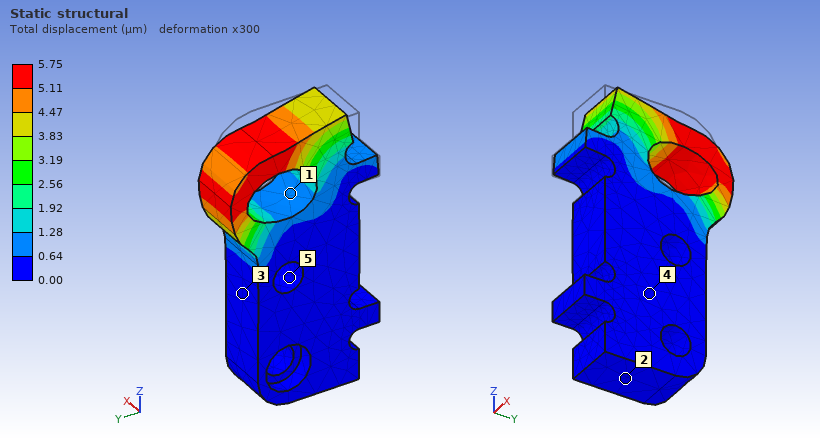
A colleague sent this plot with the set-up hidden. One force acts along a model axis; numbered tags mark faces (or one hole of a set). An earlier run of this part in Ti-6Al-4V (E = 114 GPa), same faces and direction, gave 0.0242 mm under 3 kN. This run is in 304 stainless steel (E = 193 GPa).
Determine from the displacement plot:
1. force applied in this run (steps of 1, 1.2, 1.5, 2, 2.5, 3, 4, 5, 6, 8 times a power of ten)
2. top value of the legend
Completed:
1.2 kN
5.75 µm
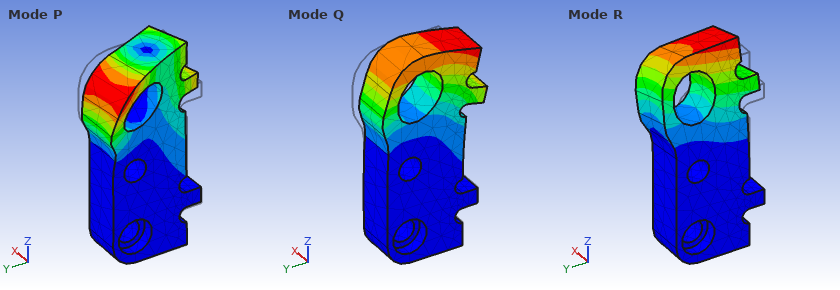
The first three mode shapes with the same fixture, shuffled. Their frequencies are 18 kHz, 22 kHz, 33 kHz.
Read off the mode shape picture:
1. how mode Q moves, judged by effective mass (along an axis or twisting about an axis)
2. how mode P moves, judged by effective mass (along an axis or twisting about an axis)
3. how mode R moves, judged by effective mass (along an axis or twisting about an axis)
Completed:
along Y
twisting about Z
along X
